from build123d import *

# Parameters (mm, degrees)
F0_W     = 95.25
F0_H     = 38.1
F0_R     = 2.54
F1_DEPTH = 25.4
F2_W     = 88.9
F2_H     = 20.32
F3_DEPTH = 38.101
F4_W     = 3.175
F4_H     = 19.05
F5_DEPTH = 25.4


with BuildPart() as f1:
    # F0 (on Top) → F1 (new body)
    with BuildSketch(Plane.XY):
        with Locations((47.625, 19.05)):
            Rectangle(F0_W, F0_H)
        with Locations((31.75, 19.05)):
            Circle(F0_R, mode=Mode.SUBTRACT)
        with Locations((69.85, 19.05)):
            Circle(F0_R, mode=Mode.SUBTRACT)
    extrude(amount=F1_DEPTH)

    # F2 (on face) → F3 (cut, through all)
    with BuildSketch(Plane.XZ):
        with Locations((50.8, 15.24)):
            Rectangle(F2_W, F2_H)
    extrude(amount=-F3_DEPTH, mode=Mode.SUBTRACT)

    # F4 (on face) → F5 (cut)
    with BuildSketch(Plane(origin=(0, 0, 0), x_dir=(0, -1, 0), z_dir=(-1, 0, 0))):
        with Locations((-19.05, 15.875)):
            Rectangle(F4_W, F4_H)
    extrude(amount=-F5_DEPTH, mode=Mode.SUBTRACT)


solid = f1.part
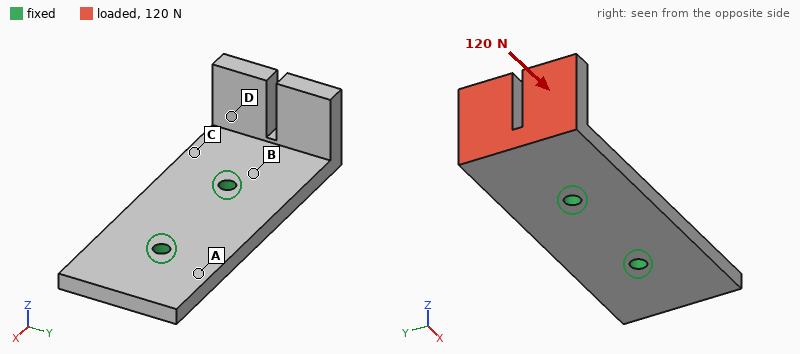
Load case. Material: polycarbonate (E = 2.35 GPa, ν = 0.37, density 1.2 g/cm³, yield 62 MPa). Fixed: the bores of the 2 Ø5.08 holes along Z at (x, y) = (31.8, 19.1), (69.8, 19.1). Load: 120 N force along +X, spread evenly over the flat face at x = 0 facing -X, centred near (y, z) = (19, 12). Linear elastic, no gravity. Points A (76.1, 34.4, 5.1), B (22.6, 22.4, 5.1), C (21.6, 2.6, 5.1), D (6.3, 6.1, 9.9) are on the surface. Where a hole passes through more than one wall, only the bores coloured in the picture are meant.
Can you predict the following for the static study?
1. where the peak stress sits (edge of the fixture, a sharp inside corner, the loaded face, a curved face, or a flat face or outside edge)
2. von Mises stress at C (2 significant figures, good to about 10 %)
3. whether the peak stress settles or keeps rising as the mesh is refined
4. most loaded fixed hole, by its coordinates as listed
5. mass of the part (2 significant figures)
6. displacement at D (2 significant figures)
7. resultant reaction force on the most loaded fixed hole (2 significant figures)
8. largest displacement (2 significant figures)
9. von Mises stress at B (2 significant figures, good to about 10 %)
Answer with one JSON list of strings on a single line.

["edge of the fixture", "7.0 MPa", "keeps rising", "(31.8, 19.1)", "27 g", "0.47 mm", "96 N", "1.1 mm", "8.2 MPa"]
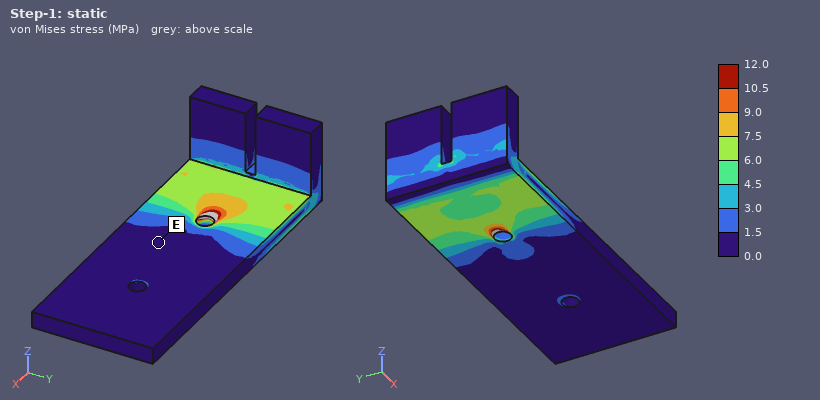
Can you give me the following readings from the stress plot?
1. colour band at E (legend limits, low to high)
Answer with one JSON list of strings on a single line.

["0.0 to 1.5 MPa"]
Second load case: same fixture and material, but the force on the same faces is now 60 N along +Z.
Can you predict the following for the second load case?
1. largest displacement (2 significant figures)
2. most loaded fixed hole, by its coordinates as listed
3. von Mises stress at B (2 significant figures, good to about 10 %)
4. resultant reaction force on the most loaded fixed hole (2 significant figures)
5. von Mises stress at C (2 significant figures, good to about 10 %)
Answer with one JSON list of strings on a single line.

["1.0 mm", "(31.8, 19.1)", "8.6 MPa", "75 N", "6.7 MPa"]
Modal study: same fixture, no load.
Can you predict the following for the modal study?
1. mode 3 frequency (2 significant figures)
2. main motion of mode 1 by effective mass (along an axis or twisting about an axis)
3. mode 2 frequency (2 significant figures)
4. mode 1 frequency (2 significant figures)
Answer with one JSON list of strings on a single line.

["1600 Hz", "along Z", "760 Hz", "520 Hz"]
